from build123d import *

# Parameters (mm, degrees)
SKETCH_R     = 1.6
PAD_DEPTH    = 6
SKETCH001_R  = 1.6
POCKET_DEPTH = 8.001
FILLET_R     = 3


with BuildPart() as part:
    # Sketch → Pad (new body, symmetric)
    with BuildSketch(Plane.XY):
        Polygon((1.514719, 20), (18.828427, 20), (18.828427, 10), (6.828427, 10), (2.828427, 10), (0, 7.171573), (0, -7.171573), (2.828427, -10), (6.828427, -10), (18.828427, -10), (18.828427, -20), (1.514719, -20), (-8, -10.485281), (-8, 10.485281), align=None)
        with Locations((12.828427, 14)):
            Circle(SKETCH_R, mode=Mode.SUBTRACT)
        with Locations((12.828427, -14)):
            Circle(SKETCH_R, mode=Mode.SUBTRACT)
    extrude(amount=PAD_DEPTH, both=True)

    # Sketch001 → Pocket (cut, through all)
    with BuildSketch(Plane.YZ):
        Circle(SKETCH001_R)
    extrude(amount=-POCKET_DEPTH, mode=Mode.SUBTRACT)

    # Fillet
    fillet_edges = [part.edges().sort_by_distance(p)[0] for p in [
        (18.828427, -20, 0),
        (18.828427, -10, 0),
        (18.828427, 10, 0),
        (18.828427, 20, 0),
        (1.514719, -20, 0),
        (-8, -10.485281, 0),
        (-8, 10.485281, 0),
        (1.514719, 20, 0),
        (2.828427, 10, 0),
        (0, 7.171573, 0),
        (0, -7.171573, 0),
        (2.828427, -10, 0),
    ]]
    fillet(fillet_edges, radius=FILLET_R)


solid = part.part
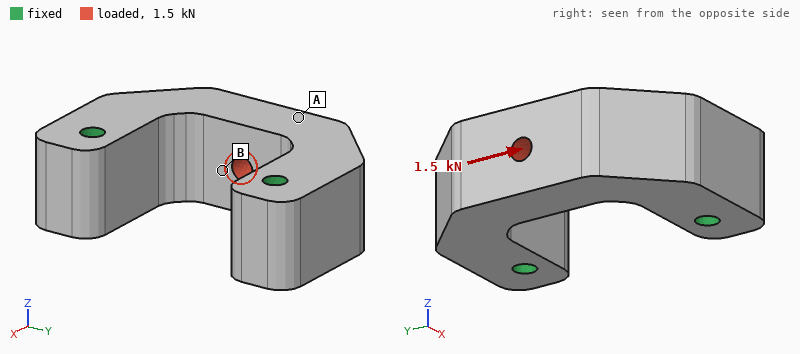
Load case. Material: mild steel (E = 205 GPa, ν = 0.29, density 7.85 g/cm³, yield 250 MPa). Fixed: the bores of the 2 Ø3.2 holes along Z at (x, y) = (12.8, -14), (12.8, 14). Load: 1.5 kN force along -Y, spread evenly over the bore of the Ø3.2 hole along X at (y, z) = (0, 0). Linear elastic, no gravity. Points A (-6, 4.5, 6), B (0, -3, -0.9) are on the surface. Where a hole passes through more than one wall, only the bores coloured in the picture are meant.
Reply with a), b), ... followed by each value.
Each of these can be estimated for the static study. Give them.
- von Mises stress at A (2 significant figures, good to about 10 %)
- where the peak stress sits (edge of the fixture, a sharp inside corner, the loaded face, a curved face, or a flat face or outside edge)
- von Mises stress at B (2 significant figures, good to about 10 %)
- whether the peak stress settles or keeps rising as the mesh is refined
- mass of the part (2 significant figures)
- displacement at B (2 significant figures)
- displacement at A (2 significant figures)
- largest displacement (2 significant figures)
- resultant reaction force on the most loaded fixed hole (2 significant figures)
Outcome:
a) 11 MPa
b) edge of the fixture
c) 24 MPa
d) keeps rising
e) 55 g
f) 5.0 µm
g) 4.6 µm
h) 5.3 µm
i) 880 N
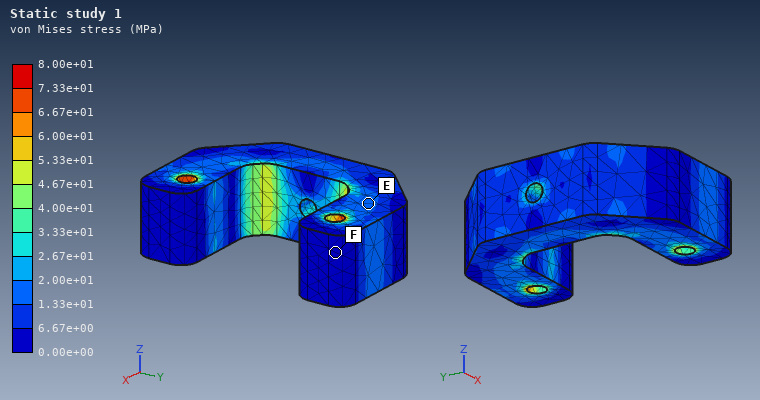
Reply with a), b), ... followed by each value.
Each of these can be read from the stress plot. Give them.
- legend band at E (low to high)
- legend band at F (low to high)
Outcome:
a) 1.33e+01 to 2.00e+01 MPa
b) 0.00e+00 to 6.67e+00 MPa
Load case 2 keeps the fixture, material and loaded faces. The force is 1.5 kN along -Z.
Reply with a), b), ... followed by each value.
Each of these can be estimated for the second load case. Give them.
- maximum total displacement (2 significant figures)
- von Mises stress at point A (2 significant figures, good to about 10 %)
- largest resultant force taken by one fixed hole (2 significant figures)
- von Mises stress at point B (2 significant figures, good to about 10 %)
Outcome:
a) 11 µm
b) 25 MPa
c) 750 N
d) 18 MPa
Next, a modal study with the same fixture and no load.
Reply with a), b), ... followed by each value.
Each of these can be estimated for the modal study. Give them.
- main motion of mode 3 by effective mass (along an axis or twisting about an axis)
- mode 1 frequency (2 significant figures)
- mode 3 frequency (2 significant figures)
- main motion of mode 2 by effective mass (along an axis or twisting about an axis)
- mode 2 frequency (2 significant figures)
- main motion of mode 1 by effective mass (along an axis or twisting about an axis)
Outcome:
a) twisting about X
b) 15 kHz
c) 27 kHz
d) along Y
e) 17 kHz
f) along Z
